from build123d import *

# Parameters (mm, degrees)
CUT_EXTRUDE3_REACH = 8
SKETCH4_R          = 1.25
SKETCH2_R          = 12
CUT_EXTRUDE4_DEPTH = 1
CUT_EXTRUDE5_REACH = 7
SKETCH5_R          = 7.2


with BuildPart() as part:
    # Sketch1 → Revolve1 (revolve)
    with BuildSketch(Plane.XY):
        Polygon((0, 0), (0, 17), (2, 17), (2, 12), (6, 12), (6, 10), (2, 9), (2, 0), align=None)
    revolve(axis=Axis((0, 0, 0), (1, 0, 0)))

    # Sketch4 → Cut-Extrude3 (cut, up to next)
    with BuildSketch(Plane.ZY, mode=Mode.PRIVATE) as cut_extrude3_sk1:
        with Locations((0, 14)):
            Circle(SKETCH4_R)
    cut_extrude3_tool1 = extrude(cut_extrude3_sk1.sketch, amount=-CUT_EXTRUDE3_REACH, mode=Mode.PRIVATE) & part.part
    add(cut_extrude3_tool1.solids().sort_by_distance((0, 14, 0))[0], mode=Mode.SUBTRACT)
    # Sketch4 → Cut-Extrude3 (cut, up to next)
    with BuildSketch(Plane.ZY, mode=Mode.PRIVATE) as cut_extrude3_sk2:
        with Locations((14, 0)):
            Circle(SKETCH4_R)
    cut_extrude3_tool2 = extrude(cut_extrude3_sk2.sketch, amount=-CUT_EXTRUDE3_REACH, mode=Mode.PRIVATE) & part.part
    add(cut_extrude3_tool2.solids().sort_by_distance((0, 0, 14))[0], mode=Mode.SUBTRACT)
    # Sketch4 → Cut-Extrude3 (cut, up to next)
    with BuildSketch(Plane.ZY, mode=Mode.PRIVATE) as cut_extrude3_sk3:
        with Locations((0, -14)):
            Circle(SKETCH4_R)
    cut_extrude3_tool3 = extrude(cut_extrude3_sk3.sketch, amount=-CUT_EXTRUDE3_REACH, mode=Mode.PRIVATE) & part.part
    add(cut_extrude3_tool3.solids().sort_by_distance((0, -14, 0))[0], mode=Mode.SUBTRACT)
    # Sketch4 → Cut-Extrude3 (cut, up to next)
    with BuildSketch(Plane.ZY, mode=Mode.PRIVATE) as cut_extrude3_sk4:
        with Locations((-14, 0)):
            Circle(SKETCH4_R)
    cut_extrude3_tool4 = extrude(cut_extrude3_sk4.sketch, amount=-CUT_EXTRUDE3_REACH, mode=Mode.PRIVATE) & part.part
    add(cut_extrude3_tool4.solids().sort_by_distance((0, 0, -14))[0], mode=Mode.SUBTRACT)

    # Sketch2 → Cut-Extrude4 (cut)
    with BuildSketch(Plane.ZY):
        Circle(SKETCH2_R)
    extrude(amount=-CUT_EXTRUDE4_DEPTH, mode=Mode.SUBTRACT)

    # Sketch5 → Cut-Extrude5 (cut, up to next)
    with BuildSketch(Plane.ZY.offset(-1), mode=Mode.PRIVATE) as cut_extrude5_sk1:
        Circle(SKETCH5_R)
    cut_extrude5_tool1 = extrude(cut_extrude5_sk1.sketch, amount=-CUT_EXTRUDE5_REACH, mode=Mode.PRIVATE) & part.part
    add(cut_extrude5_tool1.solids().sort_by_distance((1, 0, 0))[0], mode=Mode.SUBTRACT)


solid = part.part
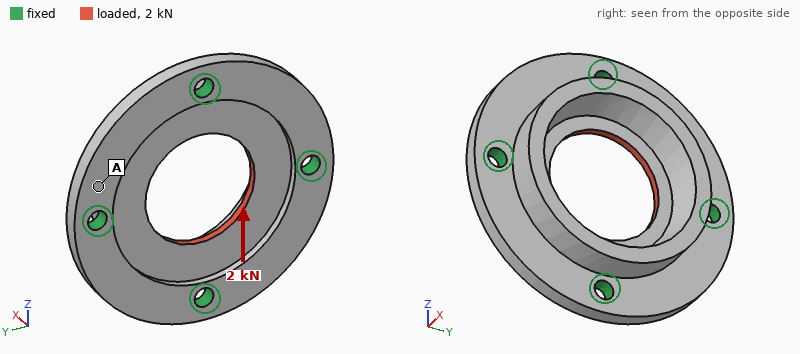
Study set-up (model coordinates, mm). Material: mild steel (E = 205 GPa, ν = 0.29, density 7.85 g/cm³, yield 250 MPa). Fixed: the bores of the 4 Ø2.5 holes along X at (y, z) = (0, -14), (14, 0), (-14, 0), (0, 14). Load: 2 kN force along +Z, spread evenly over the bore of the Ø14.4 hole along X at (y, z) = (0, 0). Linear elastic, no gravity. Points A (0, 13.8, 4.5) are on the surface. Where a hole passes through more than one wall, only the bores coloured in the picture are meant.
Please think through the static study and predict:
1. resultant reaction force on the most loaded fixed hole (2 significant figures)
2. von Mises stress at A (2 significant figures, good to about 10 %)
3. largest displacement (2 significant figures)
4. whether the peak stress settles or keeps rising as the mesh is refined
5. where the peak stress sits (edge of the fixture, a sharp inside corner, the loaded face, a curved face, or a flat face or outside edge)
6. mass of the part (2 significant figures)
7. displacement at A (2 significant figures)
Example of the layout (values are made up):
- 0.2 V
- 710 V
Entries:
- 500 N
- 20 MPa
- 2.5 µm
- keeps rising
- edge of the fixture
- 14 g
- 0.48 µm
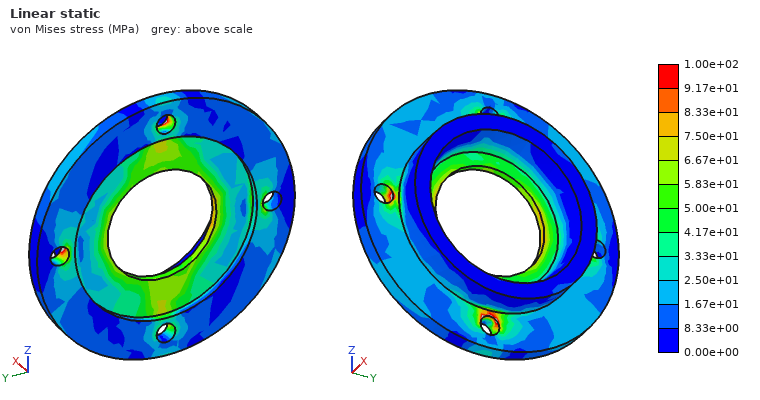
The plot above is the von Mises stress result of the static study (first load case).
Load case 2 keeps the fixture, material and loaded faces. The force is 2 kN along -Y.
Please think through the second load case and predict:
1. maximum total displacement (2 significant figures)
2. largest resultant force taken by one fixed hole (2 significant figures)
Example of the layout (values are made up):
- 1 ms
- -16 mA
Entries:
- 2.5 µm
- 500 N
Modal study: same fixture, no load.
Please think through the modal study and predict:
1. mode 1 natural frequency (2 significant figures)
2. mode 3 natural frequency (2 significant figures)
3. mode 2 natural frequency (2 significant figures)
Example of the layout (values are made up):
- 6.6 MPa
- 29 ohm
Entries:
- 23 kHz
- 27 kHz
- 26 kHz
